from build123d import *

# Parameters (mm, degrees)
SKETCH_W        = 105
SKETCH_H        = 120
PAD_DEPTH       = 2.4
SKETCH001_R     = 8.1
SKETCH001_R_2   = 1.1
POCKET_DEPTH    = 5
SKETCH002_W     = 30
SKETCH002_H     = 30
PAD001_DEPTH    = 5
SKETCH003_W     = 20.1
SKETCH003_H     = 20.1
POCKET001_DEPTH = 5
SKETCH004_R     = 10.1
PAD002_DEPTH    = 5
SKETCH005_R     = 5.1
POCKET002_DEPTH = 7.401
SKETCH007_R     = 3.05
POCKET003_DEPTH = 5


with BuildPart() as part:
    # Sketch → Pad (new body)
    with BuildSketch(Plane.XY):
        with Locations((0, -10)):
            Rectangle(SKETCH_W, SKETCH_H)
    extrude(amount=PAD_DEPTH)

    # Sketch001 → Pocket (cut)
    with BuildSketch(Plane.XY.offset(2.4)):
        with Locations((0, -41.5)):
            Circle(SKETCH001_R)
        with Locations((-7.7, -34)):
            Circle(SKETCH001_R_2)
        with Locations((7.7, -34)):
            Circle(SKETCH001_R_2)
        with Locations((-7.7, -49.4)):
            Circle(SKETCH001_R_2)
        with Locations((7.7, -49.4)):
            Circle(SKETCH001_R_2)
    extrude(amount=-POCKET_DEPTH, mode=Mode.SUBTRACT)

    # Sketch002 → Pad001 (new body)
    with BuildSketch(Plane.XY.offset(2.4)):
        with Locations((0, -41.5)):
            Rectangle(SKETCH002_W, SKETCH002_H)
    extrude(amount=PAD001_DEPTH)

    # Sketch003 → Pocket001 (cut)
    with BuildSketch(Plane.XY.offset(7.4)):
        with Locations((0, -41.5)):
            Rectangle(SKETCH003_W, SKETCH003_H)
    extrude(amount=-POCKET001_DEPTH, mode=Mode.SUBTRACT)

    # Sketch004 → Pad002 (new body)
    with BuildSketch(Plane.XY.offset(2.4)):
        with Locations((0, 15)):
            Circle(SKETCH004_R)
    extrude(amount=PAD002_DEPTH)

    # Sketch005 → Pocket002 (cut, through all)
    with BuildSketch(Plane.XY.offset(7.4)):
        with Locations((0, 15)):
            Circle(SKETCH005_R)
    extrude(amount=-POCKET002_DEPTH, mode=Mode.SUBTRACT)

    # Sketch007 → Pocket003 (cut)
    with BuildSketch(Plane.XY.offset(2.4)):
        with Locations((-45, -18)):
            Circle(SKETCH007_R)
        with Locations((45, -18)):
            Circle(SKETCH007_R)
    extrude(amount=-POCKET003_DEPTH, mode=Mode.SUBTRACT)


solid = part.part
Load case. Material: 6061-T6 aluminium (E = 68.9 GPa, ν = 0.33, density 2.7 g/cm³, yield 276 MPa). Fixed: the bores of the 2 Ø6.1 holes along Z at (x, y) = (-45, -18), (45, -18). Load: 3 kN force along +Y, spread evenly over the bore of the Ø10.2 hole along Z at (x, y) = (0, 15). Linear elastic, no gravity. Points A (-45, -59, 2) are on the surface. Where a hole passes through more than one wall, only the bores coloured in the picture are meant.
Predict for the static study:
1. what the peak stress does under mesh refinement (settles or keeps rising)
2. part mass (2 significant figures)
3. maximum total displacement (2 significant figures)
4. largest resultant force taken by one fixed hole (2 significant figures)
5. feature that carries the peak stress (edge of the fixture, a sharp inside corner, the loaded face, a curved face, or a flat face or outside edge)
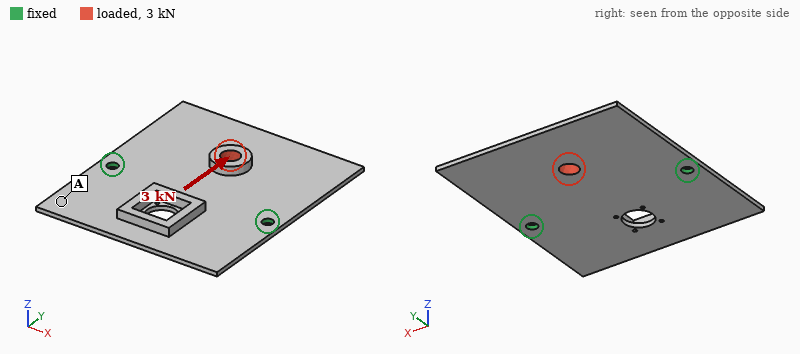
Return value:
keeps rising
89 g
1.8 mm
1.5 kN
edge of the fixture
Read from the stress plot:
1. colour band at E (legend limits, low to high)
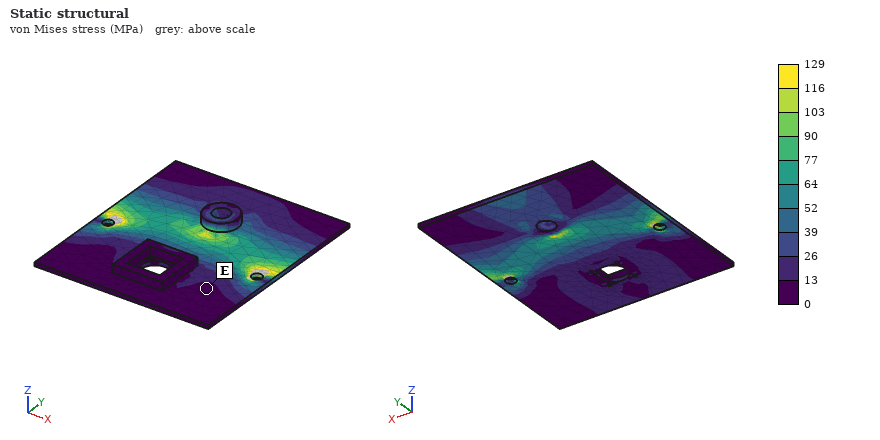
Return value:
0 to 13 MPa
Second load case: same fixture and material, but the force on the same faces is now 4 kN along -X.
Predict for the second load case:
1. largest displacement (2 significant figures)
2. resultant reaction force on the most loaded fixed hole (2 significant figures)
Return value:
0.49 mm
2.5 kN
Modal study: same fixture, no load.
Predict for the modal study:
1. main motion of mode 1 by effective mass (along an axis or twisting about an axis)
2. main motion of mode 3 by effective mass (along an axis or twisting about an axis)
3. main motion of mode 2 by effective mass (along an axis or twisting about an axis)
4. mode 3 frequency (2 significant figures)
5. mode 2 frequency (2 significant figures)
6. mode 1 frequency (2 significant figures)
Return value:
along Z
twisting about Y
along Z
840 Hz
650 Hz
350 Hz
